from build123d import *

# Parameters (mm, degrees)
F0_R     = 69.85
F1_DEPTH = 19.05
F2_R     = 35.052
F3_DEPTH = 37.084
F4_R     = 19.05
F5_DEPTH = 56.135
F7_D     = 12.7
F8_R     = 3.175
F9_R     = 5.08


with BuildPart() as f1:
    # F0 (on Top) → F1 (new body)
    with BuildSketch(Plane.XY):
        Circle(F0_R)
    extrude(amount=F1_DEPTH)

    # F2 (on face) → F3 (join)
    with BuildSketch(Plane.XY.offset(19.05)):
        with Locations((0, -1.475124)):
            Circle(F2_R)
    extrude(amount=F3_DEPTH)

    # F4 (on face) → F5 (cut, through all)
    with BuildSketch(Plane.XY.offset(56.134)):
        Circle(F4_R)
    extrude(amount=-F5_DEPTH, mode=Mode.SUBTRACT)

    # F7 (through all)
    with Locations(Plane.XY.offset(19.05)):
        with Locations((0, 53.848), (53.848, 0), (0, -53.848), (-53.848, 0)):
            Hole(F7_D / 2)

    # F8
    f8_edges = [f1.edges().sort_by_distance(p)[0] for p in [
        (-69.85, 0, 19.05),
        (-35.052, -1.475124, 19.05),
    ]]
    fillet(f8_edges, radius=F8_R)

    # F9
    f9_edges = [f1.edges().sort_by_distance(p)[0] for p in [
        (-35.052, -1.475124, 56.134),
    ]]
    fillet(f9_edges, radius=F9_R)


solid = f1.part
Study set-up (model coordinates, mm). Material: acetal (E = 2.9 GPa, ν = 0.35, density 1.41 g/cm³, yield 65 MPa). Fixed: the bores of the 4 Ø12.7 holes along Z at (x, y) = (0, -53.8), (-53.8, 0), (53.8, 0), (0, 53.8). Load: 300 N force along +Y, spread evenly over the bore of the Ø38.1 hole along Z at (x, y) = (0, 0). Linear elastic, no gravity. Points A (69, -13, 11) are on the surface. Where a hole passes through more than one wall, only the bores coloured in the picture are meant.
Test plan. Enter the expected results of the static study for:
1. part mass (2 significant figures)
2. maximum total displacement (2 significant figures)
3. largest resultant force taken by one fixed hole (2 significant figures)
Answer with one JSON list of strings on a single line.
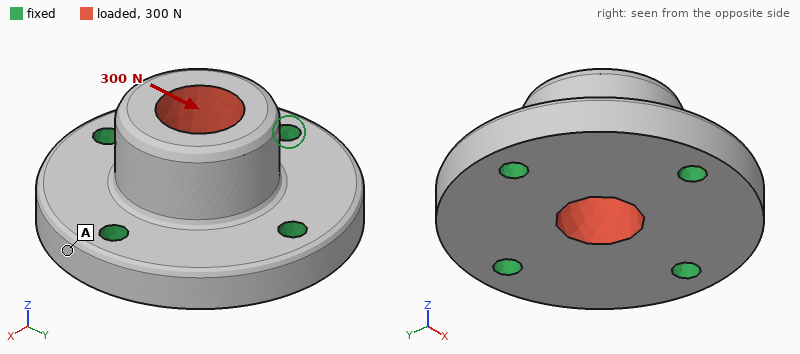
["510 g", "6.7 µm", "110 N"]
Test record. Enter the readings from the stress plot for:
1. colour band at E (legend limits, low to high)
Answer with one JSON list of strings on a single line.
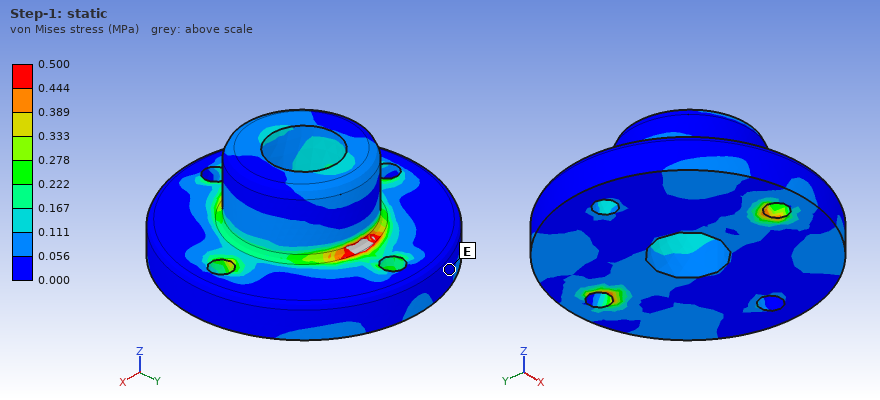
["0.000 to 0.056 MPa"]
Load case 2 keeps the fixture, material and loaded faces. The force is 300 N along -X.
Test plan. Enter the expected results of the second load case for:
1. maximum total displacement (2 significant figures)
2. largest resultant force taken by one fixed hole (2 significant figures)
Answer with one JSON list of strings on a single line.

["6.5 µm", "110 N"]
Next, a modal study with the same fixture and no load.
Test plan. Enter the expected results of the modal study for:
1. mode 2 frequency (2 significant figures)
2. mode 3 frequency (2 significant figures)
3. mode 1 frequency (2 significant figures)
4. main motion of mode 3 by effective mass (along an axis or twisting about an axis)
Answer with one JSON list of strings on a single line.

["2500 Hz", "2700 Hz", "2500 Hz", "along Z"]
